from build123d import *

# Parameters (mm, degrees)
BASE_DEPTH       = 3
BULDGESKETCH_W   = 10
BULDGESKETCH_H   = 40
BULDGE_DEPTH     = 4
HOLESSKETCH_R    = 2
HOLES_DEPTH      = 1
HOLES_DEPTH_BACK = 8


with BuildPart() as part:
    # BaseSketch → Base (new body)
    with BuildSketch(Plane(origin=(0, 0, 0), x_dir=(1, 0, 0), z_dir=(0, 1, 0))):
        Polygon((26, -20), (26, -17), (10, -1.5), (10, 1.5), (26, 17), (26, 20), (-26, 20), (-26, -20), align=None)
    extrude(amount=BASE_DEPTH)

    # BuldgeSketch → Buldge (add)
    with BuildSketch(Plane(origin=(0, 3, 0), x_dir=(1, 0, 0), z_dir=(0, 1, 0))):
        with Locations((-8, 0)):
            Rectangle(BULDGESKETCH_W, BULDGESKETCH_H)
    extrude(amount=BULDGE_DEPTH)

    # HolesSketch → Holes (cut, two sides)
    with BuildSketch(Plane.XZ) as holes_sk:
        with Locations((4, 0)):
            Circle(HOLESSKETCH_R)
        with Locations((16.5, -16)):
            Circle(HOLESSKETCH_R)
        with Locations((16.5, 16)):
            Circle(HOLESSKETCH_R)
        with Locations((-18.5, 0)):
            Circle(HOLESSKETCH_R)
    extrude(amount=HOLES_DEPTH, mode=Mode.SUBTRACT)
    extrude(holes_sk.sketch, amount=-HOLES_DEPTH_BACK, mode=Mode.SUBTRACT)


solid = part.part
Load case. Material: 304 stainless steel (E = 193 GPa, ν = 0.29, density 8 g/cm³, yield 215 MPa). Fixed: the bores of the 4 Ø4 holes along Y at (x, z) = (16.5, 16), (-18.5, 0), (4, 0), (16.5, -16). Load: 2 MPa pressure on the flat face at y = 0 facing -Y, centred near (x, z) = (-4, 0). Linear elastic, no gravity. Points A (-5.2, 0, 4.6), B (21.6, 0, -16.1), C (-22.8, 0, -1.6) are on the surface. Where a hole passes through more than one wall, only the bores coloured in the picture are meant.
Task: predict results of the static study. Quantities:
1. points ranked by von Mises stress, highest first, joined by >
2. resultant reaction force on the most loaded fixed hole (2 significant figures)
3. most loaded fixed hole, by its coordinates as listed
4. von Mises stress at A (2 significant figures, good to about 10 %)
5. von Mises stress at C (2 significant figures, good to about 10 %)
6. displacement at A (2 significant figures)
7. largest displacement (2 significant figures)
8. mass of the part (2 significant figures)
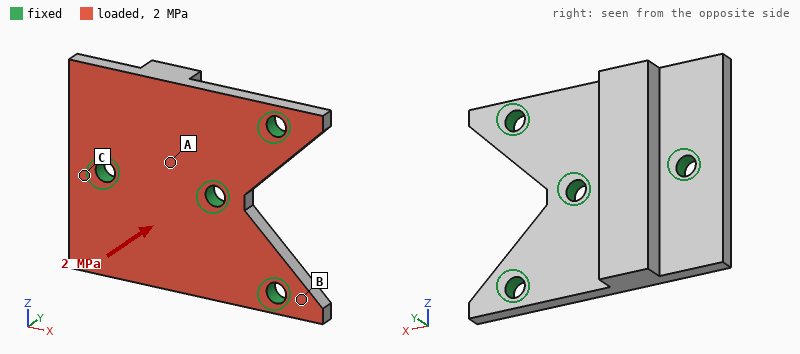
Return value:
C > A > B
1.6 kN
(-18.5, 0)
45 MPa
79 MPa
6.1 µm
31 µm
54 g
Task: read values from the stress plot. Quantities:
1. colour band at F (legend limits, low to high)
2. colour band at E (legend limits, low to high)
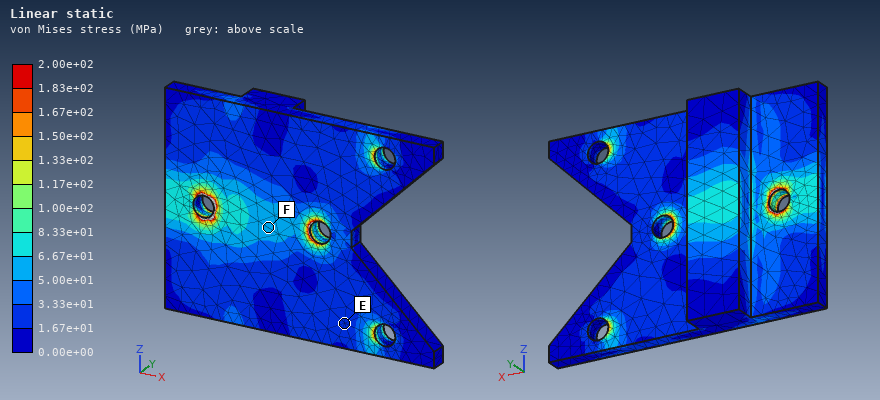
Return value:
5.00e+01 to 6.67e+01 MPa
1.67e+01 to 3.33e+01 MPa
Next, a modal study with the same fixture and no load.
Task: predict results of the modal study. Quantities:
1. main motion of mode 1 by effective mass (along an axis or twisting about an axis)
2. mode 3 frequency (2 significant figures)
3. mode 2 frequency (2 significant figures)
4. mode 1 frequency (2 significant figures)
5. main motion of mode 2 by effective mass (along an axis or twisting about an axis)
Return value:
twisting about X
15 kHz
10 kHz
6600 Hz
along Y
